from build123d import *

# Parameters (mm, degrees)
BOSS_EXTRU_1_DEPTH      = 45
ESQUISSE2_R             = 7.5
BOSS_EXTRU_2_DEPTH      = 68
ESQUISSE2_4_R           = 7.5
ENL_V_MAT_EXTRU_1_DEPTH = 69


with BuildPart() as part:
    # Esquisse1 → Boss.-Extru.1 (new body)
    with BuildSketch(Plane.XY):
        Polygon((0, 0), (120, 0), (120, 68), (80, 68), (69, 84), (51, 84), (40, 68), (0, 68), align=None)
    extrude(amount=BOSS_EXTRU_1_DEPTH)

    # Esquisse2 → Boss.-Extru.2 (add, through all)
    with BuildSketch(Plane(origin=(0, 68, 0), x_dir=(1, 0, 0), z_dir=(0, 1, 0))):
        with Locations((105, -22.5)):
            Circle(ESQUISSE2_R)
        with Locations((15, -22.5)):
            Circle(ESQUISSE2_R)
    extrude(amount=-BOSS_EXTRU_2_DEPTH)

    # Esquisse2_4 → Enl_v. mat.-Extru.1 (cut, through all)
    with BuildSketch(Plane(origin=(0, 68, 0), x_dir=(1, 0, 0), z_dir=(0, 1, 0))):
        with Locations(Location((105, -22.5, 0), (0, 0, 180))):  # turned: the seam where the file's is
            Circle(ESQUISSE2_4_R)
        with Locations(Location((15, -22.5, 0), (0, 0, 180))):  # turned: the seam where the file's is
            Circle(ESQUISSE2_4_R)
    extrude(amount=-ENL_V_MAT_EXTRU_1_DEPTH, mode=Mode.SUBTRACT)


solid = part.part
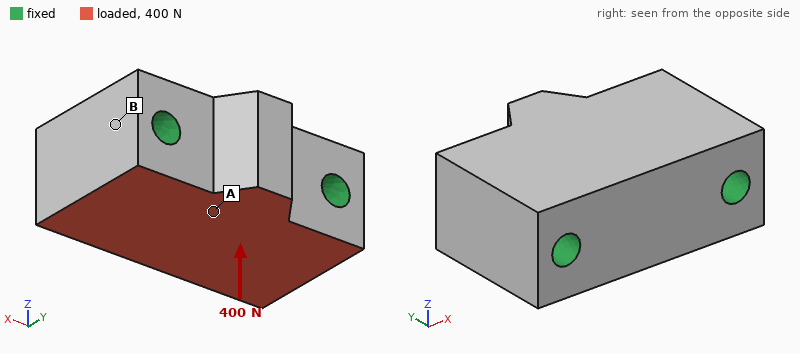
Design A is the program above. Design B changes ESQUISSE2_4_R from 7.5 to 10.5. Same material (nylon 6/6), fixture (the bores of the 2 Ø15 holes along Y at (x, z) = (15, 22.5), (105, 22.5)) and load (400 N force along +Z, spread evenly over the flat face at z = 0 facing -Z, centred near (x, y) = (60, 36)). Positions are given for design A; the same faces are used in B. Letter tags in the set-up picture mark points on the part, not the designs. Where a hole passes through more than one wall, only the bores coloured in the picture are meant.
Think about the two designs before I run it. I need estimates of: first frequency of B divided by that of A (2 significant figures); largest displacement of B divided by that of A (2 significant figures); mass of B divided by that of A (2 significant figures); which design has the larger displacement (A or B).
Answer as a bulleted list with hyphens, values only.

- 1.1
- 0.84
- 0.94
- A
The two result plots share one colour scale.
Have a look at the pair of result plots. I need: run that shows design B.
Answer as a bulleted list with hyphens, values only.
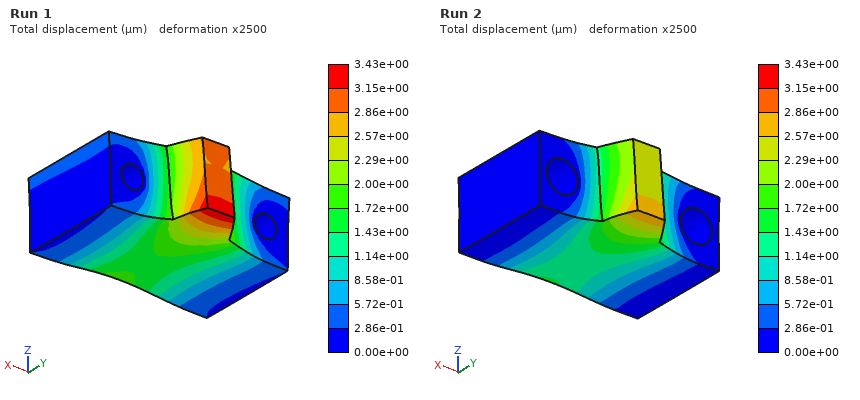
- Run 2
